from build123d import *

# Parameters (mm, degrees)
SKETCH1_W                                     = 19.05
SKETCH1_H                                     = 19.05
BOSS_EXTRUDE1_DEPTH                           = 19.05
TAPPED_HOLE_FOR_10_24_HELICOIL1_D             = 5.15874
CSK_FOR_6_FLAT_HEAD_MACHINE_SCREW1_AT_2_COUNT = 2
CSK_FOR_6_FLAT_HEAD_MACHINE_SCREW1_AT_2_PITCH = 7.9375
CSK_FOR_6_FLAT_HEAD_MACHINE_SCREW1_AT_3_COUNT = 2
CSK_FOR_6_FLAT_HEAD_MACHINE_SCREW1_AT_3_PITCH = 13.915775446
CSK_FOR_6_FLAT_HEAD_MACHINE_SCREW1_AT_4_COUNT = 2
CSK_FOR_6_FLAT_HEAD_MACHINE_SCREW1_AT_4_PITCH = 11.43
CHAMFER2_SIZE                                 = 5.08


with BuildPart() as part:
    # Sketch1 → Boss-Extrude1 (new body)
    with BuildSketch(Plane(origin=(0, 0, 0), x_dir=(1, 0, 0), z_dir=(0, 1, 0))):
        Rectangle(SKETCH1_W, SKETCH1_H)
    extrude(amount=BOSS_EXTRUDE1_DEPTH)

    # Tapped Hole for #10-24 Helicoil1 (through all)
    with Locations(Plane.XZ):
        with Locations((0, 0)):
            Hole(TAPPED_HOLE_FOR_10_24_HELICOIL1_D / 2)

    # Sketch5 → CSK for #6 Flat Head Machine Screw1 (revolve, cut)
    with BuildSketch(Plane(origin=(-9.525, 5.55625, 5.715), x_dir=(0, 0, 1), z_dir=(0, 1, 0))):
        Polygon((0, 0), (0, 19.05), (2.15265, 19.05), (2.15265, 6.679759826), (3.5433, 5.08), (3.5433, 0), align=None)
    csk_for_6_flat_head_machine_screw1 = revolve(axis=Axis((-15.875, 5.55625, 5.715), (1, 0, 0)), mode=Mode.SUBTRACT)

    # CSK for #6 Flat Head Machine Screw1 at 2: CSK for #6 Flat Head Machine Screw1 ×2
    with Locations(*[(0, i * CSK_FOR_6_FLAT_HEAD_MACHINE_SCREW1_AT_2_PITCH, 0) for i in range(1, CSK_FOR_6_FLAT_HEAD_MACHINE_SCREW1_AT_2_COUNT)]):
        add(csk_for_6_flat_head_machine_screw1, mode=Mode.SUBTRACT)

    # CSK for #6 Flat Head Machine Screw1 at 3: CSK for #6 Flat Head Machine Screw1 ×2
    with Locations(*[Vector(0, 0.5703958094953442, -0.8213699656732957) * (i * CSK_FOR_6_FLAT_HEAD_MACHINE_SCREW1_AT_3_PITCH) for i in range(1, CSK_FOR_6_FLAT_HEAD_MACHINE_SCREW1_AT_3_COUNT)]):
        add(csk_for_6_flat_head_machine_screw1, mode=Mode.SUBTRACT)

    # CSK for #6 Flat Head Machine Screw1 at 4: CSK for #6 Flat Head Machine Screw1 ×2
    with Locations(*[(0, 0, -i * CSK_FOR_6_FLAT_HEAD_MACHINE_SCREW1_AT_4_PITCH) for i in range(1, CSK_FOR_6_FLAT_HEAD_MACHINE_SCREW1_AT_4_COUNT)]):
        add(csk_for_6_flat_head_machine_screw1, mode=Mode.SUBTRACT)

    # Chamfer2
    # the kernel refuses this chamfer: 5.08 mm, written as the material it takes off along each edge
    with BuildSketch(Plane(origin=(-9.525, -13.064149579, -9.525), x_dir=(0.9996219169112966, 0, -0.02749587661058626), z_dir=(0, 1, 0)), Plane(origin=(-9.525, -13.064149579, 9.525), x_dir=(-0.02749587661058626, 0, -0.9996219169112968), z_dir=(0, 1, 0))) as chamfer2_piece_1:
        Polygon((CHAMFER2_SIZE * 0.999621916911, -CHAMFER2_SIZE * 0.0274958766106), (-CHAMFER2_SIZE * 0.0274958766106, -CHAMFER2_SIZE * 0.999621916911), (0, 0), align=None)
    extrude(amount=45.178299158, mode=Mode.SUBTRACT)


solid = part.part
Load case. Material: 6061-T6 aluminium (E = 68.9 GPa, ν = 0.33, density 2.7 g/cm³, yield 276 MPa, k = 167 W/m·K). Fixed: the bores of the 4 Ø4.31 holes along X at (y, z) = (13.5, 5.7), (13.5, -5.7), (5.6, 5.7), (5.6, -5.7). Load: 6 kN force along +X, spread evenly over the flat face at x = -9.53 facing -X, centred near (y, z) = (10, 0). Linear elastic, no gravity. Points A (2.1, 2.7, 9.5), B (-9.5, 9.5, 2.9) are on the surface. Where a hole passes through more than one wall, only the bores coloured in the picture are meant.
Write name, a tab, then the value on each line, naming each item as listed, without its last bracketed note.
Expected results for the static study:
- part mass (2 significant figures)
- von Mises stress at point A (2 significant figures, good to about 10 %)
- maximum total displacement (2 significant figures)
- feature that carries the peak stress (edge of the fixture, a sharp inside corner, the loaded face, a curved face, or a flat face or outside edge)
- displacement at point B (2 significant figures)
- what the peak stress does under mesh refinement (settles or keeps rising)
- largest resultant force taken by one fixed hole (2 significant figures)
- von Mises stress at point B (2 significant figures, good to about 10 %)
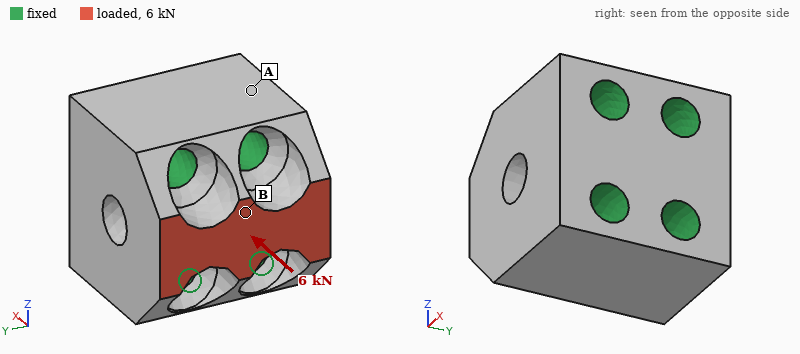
part mass	12 g
von Mises stress at point A	12 MPa
maximum total displacement	8.7 µm
feature that carries the peak stress	edge of the fixture
displacement at point B	6.4 µm
what the peak stress does under mesh refinement	keeps rising
largest resultant force taken by one fixed hole	1.7 kN
von Mises stress at point B	50 MPa
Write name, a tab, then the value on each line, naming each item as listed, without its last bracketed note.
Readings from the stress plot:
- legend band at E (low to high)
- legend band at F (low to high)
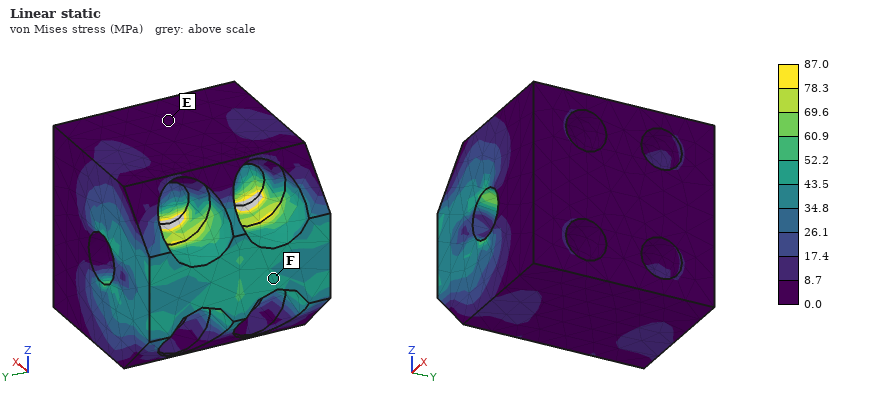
legend band at E	0.0 to 8.7 MPa
legend band at F	43.5 to 52.2 MPa
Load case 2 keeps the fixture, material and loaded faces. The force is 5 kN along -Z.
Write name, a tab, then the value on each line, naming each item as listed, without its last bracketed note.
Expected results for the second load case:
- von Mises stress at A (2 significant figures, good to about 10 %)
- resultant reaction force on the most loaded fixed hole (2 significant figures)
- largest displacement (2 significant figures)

von Mises stress at A	24 MPa
resultant reaction force on the most loaded fixed hole	2.1 kN
largest displacement	21 µm
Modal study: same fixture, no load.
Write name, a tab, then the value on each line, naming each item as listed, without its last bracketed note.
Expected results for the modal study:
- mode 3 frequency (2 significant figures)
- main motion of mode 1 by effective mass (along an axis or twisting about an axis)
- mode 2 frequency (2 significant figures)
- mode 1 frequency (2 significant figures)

mode 3 frequency	86 kHz
main motion of mode 1 by effective mass	along Y
mode 2 frequency	84 kHz
mode 1 frequency	61 kHz
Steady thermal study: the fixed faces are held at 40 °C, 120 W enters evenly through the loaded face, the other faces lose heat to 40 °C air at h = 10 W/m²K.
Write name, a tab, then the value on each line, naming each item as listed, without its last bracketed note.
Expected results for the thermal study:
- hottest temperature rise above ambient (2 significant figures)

hottest temperature rise above ambient	45 K
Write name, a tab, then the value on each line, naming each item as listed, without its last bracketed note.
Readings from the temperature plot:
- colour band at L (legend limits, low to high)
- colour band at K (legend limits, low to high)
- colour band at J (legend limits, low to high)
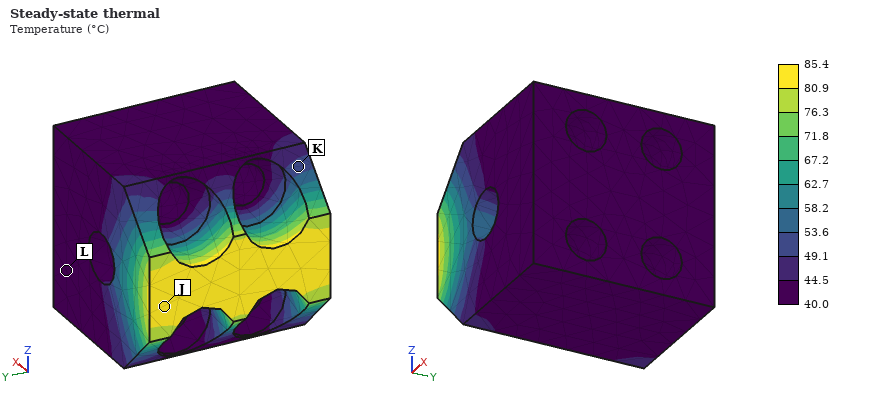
colour band at L	40.0 to 44.5 °C
colour band at K	49.1 to 53.6 °C
colour band at J	80.9 to 85.4 °C
